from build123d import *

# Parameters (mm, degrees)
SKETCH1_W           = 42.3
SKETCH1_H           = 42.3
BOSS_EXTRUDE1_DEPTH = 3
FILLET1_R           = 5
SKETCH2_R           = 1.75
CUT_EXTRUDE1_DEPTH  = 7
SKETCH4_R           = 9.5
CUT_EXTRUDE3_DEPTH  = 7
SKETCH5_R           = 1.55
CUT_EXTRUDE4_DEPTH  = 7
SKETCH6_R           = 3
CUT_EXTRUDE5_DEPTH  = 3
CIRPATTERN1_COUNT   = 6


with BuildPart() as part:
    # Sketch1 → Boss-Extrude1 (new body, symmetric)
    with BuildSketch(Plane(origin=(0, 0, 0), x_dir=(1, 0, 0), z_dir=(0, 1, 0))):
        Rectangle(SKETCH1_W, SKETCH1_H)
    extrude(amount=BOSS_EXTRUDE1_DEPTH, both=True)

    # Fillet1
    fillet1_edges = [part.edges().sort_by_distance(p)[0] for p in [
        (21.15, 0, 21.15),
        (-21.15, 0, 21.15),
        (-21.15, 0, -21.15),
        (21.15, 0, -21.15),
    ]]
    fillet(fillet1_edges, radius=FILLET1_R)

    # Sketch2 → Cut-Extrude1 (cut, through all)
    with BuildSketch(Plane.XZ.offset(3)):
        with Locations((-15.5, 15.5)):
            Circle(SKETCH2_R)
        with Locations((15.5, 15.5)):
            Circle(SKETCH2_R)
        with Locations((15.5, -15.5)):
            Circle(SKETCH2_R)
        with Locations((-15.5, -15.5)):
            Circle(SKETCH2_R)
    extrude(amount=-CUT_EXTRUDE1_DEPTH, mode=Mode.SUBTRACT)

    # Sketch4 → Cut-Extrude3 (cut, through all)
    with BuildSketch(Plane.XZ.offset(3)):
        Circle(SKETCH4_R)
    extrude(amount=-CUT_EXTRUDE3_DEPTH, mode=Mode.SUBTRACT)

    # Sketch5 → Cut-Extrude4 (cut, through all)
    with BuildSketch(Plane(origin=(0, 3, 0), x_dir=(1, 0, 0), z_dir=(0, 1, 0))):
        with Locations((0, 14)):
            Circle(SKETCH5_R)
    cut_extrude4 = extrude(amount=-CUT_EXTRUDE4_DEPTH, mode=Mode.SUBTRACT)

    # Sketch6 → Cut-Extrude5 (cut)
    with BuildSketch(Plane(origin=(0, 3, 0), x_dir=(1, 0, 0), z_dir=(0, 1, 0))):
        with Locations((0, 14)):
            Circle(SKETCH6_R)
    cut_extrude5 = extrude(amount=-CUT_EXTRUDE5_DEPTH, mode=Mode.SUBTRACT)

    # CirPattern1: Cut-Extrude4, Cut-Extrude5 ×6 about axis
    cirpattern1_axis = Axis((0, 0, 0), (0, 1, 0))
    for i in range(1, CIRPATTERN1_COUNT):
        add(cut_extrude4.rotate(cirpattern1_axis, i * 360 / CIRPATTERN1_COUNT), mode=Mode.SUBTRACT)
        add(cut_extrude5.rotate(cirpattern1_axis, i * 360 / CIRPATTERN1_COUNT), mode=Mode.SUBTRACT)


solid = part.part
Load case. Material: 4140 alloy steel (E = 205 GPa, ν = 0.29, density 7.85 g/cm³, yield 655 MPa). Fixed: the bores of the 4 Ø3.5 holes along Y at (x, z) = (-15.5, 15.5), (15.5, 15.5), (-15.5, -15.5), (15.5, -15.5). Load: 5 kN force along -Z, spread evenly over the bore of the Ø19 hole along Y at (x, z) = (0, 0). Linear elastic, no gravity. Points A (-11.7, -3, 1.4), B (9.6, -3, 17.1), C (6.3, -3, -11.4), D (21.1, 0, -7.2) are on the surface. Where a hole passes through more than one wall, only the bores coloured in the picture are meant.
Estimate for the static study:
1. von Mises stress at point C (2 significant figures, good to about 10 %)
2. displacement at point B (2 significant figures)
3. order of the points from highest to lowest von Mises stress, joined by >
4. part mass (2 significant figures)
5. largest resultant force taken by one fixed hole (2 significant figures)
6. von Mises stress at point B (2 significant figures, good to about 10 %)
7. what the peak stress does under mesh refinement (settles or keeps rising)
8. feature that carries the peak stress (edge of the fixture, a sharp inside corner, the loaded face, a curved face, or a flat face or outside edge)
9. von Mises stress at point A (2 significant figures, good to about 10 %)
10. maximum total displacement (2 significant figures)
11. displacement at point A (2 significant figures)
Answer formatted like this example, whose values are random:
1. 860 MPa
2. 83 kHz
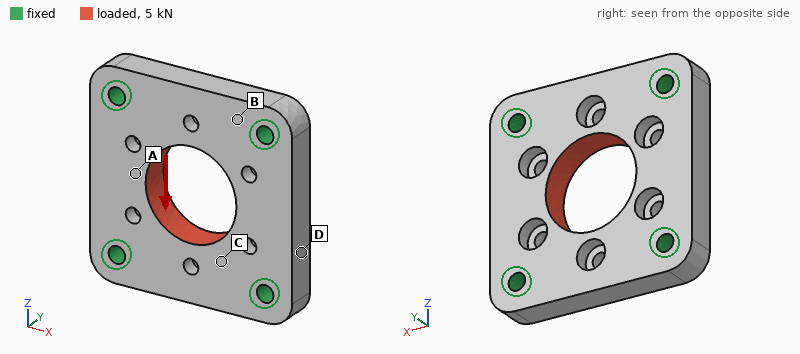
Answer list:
1. 13 MPa
2. 1.2 µm
3. A > B > C > D
4. 63 g
5. 1.3 kN
6. 19 MPa
7. keeps rising
8. edge of the fixture
9. 26 MPa
10. 3.3 µm
11. 1.5 µm
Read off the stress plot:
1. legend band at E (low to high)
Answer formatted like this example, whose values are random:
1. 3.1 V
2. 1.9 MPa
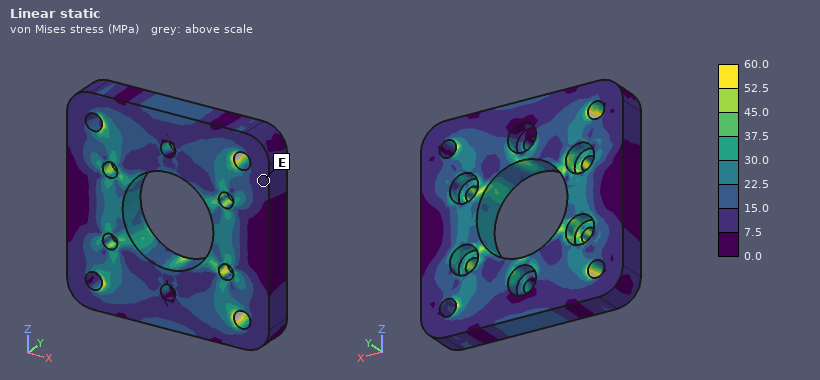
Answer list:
1. 7.5 to 15.0 MPa
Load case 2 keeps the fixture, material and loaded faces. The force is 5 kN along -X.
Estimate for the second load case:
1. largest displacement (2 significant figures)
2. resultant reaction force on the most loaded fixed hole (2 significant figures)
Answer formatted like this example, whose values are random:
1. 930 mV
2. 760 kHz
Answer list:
1. 3.3 µm
2. 1.3 kN
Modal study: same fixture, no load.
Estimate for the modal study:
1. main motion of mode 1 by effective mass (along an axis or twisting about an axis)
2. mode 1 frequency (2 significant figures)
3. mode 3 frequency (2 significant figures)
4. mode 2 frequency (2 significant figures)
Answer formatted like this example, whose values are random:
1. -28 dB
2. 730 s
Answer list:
1. along Y
2. 24 kHz
3. 28 kHz
4. 28 kHz
